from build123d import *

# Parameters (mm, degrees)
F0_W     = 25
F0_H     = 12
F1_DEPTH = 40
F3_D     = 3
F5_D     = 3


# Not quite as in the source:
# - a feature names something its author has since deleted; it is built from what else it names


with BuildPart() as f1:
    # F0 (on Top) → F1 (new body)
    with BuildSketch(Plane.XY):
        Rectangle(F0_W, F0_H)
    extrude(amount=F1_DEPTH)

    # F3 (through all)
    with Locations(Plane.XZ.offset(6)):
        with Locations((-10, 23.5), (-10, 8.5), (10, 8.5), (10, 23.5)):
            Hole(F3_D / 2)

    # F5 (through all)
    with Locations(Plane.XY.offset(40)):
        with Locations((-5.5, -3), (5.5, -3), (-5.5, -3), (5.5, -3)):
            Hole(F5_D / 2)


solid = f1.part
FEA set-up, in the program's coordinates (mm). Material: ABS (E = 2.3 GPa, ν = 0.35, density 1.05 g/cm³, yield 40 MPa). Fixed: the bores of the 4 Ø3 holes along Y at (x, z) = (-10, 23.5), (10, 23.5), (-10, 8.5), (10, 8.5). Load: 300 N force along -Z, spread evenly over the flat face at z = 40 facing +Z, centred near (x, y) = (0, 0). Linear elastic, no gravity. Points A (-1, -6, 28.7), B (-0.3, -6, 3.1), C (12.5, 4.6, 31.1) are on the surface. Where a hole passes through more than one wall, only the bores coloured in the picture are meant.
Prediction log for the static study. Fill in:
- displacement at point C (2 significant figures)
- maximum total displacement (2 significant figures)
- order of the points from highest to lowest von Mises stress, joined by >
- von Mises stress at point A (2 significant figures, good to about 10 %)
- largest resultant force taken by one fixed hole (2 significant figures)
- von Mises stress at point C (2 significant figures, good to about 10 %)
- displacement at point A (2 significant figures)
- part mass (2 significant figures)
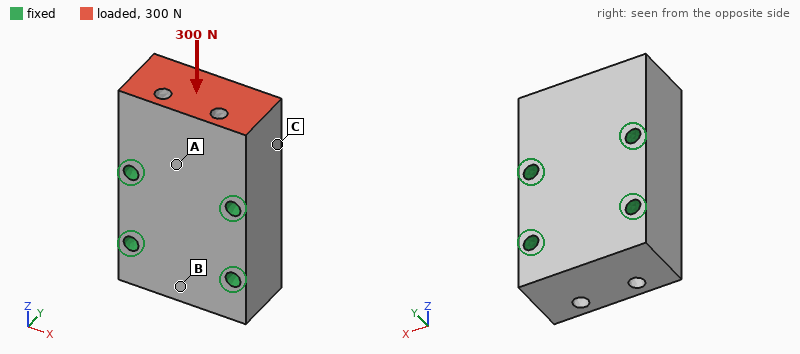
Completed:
4.3 µm
8.9 µm
C > A > B
0.65 MPa
130 N
1.2 MPa
4.6 µm
12 g
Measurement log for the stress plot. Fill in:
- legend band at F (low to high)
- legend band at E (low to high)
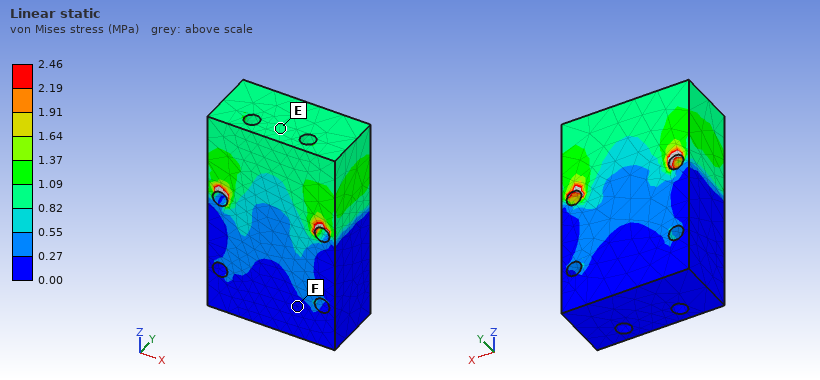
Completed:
0.00 to 0.27 MPa
0.82 to 1.09 MPa
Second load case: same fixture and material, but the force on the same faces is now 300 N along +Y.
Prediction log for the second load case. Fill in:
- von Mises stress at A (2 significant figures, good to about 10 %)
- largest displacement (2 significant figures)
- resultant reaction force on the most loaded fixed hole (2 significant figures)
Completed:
4.2 MPa
0.11 mm
180 N
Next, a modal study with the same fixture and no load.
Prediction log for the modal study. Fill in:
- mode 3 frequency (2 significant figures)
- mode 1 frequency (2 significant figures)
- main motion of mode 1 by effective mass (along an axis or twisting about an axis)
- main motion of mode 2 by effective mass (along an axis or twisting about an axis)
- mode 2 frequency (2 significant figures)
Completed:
11 kHz
7000 Hz
along Y
along X
11 kHz
